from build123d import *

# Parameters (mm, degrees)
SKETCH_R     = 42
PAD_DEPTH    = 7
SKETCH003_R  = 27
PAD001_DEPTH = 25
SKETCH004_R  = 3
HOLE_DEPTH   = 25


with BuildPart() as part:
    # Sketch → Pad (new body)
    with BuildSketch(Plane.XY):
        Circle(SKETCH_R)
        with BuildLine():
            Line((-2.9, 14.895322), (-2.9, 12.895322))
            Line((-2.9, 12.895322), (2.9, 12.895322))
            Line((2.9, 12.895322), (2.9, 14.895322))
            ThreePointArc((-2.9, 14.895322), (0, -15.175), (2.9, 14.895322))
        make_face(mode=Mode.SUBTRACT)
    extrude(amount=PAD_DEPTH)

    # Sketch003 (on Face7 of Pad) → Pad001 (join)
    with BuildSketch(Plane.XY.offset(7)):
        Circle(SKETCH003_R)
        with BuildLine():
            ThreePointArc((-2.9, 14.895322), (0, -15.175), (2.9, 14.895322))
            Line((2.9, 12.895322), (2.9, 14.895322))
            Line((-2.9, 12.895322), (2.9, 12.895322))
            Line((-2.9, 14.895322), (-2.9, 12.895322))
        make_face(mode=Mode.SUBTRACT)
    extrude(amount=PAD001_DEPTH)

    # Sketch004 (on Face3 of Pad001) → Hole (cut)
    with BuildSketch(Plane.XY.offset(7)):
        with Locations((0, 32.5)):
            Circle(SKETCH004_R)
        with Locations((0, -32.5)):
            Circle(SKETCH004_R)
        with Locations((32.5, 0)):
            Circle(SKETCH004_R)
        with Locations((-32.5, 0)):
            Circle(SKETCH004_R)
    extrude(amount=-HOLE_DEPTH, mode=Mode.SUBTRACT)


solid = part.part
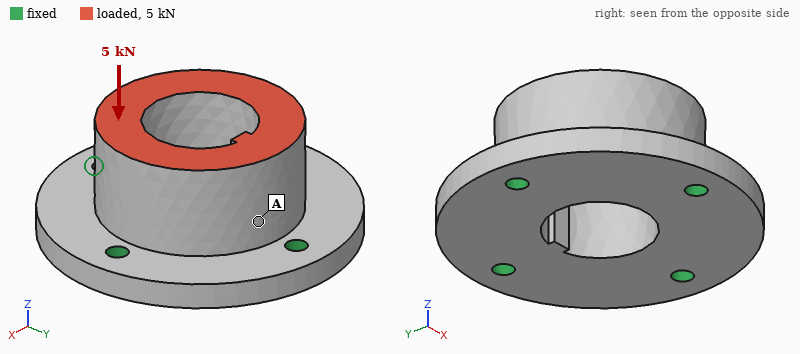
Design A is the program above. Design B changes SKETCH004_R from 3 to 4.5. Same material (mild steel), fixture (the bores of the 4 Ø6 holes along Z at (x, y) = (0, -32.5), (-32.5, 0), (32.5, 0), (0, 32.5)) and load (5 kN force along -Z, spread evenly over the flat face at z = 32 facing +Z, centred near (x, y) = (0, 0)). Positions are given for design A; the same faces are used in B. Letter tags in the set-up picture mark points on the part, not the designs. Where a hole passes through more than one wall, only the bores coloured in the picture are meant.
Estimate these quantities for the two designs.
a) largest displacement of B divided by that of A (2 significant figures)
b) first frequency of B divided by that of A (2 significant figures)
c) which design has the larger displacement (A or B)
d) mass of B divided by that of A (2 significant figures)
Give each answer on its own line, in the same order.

0.73
1.2
A
0.99
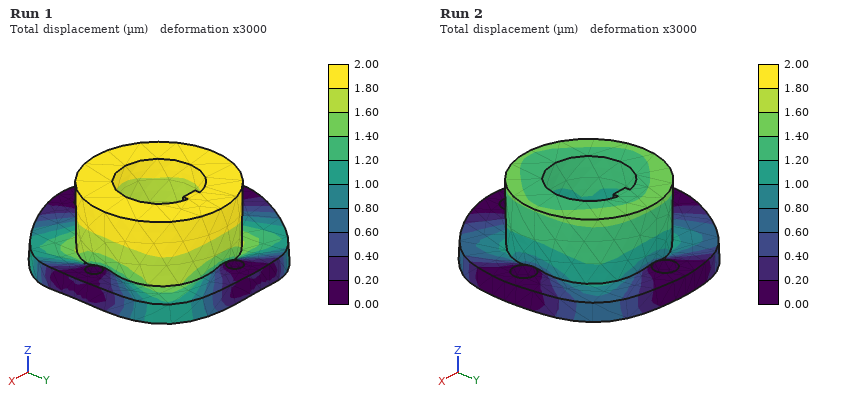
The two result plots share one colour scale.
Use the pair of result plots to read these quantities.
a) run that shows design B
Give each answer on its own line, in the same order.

Run 2
